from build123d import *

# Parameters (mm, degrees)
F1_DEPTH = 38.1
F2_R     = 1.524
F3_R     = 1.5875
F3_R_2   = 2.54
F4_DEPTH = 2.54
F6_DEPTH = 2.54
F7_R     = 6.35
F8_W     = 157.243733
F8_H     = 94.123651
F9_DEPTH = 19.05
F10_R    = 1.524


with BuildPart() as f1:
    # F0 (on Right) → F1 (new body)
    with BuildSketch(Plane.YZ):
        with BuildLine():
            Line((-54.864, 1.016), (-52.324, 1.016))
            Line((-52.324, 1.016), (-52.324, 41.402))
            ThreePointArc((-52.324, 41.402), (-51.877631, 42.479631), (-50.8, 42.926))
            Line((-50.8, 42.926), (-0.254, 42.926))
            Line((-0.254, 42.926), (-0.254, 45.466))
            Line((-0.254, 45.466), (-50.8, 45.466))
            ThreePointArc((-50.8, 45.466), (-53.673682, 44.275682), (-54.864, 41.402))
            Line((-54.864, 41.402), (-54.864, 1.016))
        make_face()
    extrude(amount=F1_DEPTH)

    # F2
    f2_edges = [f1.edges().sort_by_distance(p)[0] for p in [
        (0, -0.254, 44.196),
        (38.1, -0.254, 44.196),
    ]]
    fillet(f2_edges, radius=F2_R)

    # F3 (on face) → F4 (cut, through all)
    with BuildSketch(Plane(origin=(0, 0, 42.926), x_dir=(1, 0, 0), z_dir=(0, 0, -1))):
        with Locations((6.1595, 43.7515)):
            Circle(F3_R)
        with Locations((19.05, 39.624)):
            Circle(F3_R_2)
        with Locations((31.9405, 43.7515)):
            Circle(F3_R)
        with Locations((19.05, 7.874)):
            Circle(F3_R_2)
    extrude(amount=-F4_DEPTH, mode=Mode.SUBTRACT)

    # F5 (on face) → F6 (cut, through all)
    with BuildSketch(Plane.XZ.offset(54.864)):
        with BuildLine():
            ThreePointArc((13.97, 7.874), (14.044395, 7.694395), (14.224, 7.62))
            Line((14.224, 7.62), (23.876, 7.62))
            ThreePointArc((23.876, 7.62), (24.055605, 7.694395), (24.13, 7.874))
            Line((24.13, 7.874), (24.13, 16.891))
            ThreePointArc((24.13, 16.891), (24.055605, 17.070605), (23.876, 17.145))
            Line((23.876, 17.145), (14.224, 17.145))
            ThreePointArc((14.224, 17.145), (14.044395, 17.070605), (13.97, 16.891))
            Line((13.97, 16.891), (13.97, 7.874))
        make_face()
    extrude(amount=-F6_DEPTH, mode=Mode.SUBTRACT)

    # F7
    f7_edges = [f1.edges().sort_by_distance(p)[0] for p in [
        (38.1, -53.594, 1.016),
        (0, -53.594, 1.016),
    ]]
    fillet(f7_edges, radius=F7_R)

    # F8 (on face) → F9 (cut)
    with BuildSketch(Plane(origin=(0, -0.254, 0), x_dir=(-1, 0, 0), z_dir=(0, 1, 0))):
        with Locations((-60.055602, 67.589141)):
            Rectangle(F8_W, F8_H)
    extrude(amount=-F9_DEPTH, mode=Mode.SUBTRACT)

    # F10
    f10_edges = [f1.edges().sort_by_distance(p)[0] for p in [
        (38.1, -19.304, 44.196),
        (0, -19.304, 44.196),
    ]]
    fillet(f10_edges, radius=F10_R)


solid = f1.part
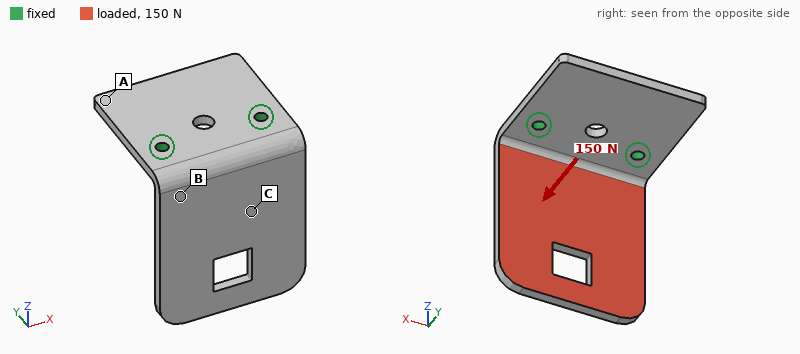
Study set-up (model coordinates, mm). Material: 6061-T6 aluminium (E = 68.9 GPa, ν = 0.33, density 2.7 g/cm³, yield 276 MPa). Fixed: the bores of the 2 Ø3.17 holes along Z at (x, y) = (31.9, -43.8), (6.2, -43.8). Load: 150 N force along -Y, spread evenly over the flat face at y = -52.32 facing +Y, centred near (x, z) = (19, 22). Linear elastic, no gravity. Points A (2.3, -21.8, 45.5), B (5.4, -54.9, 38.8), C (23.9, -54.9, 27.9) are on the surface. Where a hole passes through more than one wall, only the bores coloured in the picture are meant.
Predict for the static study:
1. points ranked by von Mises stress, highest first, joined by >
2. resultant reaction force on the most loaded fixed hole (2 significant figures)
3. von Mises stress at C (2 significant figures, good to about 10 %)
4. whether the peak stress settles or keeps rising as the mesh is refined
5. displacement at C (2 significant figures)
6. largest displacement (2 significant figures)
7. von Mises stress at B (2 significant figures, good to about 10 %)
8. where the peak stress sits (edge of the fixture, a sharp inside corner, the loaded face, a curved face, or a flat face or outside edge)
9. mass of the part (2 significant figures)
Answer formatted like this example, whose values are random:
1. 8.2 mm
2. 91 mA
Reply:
1. B > C > A
2. 78 N
3. 26 MPa
4. keeps rising
5. 0.23 mm
6. 0.75 mm
7. 55 MPa
8. edge of the fixture
9. 19 g
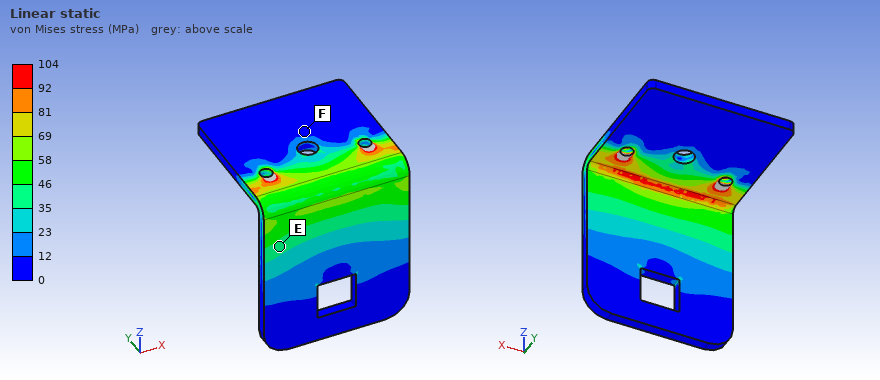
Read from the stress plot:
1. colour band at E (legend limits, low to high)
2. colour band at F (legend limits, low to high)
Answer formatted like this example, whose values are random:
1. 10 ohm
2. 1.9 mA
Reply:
1. 35 to 46 MPa
2. 0 to 12 MPa
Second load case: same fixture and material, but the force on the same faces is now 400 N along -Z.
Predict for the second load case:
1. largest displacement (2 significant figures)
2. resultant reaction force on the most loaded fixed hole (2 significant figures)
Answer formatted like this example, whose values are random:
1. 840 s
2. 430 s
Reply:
1. 0.11 mm
2. 200 N
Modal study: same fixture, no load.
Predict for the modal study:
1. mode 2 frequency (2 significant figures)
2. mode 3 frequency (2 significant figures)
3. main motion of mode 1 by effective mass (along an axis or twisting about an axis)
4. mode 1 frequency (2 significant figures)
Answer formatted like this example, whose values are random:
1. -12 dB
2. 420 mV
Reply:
1. 2500 Hz
2. 3300 Hz
3. along Y
4. 900 Hz
